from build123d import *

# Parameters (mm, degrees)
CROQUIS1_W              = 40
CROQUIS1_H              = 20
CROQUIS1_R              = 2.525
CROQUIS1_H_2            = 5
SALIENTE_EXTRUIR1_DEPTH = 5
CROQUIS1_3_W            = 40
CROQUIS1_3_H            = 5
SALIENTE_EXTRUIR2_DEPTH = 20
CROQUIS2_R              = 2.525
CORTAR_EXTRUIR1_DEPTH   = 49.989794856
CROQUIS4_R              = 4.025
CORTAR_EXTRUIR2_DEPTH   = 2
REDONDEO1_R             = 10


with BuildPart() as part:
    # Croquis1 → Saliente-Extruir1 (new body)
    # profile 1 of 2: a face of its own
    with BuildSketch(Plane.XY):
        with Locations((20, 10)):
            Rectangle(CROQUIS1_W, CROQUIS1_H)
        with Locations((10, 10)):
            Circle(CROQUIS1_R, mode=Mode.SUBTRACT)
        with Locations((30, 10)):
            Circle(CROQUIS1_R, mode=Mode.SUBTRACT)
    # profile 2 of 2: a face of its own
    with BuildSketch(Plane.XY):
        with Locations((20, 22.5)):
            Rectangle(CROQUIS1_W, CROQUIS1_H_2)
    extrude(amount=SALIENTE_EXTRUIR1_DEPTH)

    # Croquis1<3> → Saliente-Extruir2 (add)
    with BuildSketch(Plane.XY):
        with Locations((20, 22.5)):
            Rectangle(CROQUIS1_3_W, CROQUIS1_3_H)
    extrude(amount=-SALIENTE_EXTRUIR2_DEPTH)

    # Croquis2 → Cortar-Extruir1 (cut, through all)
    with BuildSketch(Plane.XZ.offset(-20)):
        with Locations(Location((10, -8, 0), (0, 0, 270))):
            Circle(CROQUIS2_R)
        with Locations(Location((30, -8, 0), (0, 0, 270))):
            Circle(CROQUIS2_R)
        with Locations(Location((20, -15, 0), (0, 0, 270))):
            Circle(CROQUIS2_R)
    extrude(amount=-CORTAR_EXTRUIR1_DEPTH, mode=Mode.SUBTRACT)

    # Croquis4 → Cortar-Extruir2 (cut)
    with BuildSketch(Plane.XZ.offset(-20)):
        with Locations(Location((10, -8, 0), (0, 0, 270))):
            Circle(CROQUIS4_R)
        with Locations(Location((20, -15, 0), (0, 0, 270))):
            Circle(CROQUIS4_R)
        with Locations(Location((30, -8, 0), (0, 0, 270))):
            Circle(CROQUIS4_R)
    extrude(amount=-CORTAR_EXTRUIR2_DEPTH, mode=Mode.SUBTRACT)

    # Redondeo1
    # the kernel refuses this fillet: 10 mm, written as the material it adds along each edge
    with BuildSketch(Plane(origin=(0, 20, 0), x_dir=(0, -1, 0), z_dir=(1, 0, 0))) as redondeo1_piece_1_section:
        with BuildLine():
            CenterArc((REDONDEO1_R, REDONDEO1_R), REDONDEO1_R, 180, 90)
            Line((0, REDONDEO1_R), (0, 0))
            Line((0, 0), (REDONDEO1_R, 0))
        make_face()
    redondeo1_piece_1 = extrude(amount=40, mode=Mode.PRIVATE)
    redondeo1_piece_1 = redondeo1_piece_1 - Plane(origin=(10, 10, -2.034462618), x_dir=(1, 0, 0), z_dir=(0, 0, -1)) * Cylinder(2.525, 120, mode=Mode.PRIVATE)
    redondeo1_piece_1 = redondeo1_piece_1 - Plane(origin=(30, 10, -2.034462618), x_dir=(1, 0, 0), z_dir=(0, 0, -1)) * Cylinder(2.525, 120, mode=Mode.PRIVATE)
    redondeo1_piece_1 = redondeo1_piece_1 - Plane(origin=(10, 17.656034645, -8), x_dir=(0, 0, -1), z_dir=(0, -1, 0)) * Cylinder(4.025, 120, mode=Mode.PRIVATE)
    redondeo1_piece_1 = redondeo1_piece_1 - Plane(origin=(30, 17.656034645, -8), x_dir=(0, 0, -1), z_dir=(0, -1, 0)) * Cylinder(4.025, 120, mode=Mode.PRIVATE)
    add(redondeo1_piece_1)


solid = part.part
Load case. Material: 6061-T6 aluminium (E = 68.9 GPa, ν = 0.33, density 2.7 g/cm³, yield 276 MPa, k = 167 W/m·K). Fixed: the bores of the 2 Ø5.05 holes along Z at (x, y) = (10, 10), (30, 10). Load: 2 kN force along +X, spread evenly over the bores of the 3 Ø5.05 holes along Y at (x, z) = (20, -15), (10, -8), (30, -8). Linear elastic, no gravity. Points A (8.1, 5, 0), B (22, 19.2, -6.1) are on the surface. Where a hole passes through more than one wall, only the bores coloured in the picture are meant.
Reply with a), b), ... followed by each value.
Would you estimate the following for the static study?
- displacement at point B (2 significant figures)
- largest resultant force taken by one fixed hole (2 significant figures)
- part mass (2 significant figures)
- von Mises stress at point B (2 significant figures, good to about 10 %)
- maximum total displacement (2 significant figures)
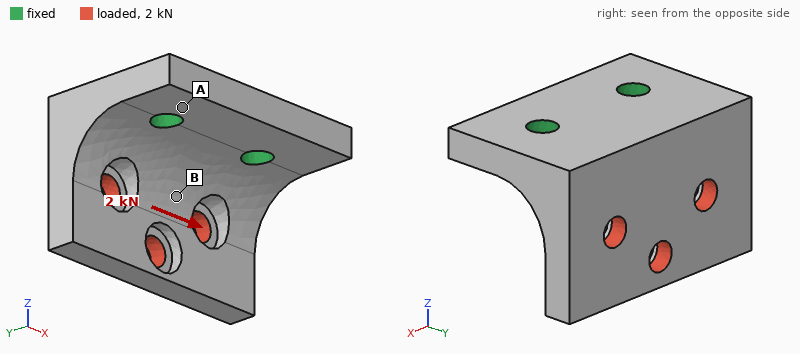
a) 14 µm
b) 1.8 kN
c) 25 g
d) 44 MPa
e) 40 µm
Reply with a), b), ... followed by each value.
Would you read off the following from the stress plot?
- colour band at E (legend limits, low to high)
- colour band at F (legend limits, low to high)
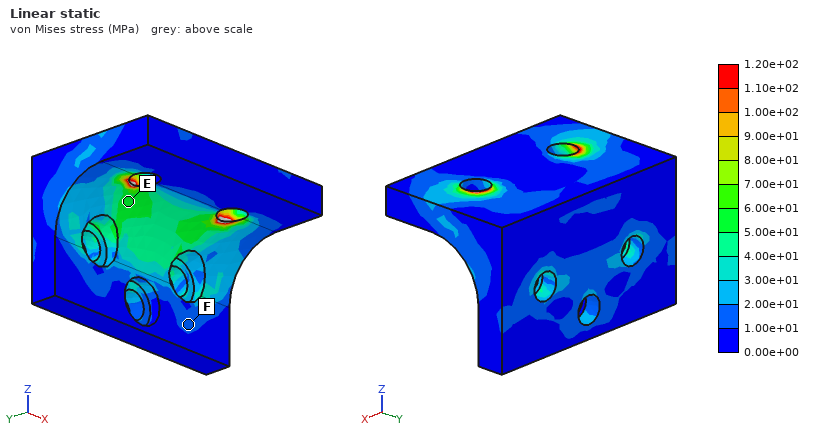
a) 5.00e+01 to 6.00e+01 MPa
b) 1.00e+01 to 2.00e+01 MPa
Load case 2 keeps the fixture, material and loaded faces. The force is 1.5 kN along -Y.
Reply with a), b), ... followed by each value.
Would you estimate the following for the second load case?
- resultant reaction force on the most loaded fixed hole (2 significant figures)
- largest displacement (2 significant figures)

a) 770 N
b) 0.12 mm
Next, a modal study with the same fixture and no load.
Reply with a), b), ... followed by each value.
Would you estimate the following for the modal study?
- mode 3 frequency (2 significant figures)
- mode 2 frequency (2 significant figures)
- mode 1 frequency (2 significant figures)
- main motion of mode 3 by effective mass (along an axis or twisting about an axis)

a) 15 kHz
b) 9900 Hz
c) 6300 Hz
d) along X
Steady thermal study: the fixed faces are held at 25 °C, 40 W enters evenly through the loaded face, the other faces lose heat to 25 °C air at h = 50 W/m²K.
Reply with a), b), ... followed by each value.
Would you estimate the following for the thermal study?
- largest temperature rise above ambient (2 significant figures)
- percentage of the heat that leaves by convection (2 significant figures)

a) 29 K
b) 5.8 %
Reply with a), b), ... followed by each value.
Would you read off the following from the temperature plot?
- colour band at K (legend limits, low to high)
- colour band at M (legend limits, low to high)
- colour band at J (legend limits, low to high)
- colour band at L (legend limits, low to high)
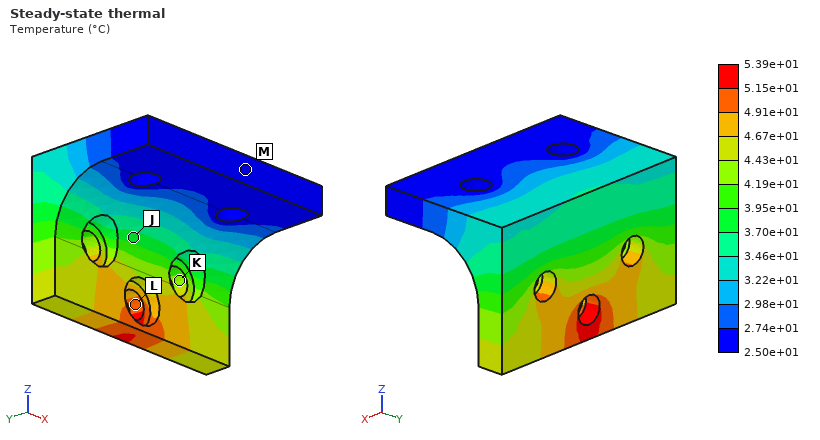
a) 4.19e+01 to 4.43e+01 °C
b) 2.50e+01 to 2.74e+01 °C
c) 3.70e+01 to 3.95e+01 °C
d) 4.91e+01 to 5.15e+01 °C
